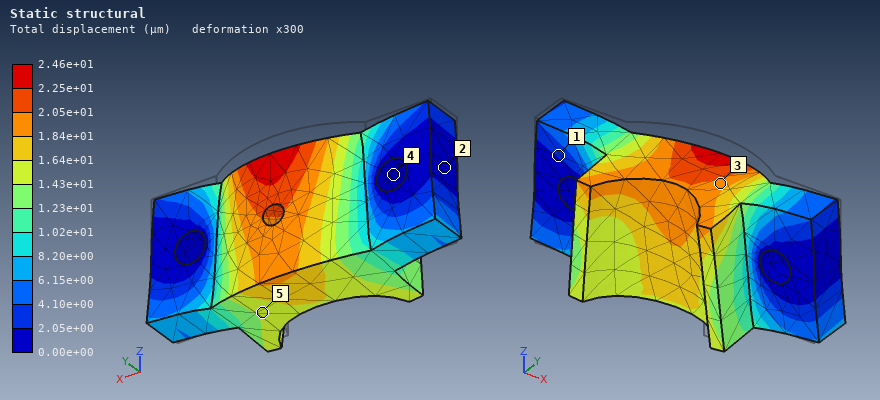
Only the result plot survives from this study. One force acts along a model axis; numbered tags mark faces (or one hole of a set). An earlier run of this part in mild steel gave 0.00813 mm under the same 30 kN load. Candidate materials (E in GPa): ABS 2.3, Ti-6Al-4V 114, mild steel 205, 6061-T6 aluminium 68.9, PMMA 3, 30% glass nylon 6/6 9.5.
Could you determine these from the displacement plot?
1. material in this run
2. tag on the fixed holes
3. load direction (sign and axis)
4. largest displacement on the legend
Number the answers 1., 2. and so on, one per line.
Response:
1. 6061-T6 aluminium
2. 4
3. -Z
4. 2.46e+01 µm
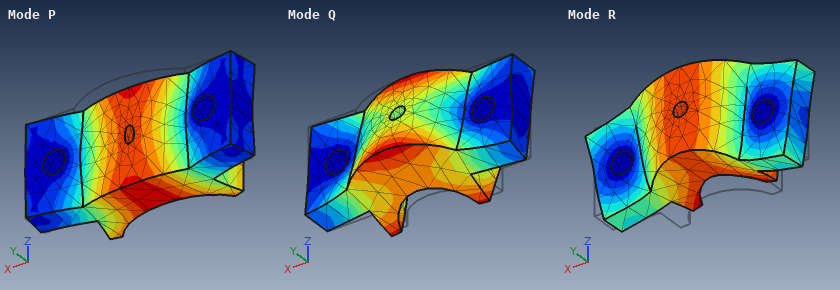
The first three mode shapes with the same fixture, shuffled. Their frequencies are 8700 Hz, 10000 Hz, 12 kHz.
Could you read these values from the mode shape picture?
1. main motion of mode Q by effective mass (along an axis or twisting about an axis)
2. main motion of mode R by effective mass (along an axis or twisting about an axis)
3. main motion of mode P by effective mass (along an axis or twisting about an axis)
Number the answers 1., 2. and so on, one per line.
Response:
1. twisting about X
2. along Z
3. along Y
